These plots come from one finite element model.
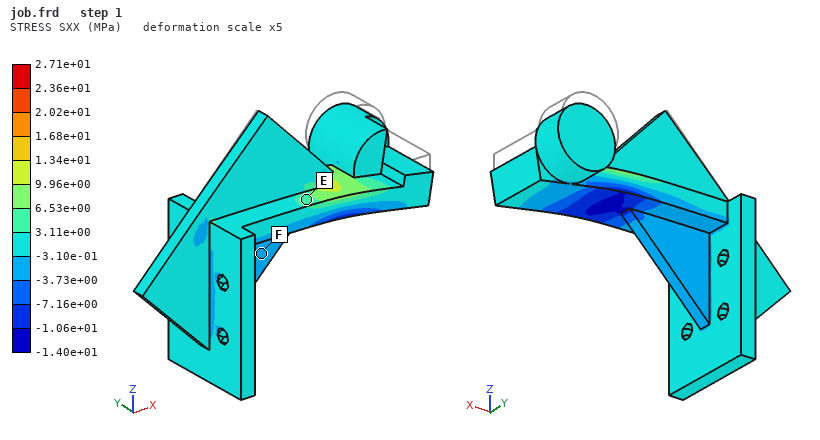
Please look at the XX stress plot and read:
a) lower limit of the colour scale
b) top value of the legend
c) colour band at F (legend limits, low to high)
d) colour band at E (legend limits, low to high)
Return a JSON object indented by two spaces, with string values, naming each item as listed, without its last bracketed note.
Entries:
{
  "lower limit of the colour scale": "-1.40e+01 MPa",
  "top value of the legend": "2.71e+01 MPa",
  "colour band at F": "-3.73e+00 to -3.10e-01 MPa",
  "colour band at E": "3.11e+00 to 6.53e+00 MPa"
}
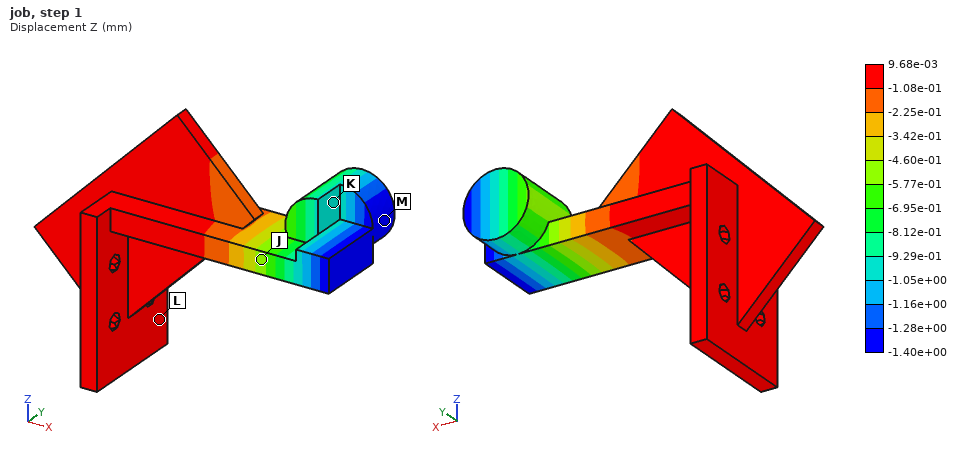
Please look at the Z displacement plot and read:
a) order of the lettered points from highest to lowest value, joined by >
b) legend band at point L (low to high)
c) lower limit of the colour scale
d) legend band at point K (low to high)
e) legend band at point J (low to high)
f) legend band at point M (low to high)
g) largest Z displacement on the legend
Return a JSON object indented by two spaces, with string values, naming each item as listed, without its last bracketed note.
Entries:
{
  "order of the lettered points from highest to lowest value, joined by >": "L > J > K > M",
  "legend band at point L": "-1.08e-01 to 9.68e-03 mm",
  "lower limit of the colour scale": "-1.40e+00 mm",
  "legend band at point K": "-1.05e+00 to -9.29e-01 mm",
  "legend band at point J": "-5.77e-01 to -4.60e-01 mm",
  "legend band at point M": "-1.40e+00 to -1.28e+00 mm",
  "largest Z displacement on the legend": "9.68e-03 mm"
}
